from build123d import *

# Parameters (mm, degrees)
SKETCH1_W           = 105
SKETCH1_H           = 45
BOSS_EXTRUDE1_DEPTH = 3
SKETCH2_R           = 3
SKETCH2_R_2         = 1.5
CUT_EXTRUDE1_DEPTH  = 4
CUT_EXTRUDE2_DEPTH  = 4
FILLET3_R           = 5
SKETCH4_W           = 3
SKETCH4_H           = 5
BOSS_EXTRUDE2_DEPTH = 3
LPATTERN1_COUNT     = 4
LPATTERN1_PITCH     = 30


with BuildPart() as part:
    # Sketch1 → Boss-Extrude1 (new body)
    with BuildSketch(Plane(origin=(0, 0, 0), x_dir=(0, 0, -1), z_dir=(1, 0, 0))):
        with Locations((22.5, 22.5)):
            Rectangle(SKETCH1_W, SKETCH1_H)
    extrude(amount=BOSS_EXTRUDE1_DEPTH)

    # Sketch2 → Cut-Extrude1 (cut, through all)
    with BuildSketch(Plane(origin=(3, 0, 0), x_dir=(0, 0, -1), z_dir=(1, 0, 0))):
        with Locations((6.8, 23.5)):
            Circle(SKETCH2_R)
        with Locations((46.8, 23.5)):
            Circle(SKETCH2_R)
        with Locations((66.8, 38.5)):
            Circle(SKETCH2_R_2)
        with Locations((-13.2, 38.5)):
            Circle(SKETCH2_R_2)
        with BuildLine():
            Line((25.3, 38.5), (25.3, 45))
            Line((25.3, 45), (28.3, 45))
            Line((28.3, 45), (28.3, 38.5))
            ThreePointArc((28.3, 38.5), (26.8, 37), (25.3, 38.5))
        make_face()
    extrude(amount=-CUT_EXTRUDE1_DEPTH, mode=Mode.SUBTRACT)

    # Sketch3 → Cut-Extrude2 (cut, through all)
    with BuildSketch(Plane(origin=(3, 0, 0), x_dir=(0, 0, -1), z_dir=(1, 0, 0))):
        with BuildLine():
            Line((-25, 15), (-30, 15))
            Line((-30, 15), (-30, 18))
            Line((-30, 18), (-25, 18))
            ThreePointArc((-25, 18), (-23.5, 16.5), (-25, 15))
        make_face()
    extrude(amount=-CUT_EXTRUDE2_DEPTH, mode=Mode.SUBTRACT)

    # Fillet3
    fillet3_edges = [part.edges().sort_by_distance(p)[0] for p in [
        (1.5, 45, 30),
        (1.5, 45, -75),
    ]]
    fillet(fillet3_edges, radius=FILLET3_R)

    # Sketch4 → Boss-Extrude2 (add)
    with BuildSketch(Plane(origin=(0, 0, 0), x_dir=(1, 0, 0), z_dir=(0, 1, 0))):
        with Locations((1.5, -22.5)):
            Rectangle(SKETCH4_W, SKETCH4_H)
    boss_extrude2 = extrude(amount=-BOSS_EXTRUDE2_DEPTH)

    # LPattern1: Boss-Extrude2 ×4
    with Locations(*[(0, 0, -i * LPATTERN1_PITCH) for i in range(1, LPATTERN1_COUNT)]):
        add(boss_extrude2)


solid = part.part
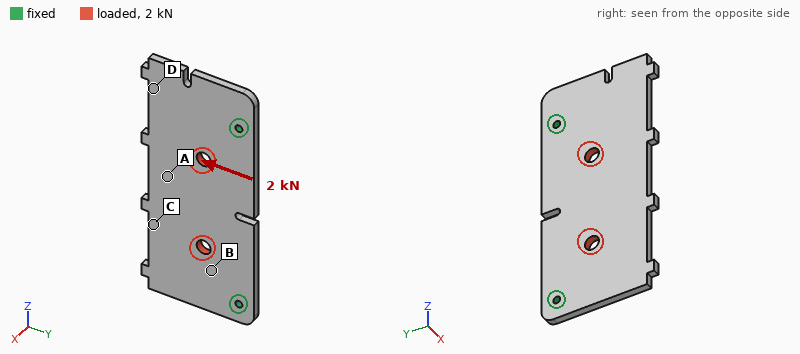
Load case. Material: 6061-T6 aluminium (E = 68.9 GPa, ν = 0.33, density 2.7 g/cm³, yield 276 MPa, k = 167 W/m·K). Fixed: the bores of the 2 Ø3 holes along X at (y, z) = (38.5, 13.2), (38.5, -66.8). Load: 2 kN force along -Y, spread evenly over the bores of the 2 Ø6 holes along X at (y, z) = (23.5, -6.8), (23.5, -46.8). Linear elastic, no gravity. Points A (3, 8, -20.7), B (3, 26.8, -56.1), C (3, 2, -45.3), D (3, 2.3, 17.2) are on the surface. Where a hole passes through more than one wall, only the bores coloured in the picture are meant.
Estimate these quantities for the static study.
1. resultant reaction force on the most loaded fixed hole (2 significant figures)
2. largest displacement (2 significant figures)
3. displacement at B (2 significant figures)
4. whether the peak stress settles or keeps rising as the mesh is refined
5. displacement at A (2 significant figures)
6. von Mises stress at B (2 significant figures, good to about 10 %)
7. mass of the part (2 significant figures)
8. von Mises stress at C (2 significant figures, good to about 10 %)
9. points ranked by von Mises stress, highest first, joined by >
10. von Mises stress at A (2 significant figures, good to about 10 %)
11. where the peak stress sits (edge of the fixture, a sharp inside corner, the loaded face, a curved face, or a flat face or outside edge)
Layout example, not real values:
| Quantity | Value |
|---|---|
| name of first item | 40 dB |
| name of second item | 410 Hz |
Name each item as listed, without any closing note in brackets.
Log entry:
| Quantity | Value |
|---|---|
| resultant reaction force on the most loaded fixed hole | 1.2 kN |
| largest displacement | 18 µm |
| displacement at B | 8.9 µm |
| whether the peak stress settles or keeps rising as the mesh is refined | keeps rising |
| displacement at A | 16 µm |
| von Mises stress at B | 20 MPa |
| mass of the part | 38 g |
| von Mises stress at C | 14 MPa |
| points ranked by von Mises stress, highest first, joined by > | B > C > A > D |
| von Mises stress at A | 11 MPa |
| where the peak stress sits | edge of the fixture |
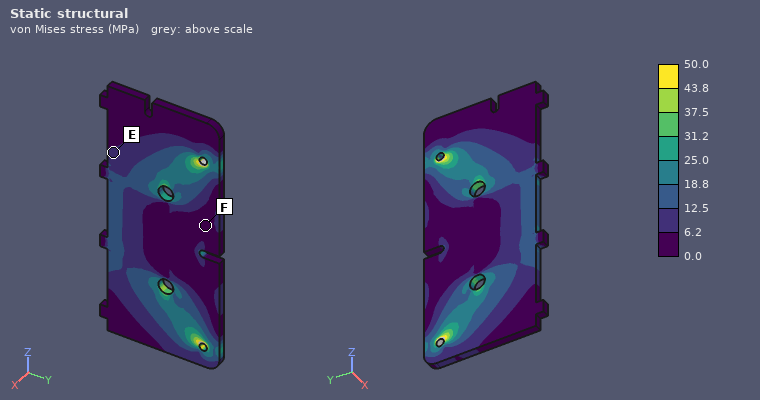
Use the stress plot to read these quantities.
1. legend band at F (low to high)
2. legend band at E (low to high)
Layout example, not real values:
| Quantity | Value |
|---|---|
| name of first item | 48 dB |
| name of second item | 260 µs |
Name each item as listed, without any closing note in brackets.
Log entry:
| Quantity | Value |
|---|---|
| legend band at F | 0.0 to 6.2 MPa |
| legend band at E | 6.2 to 12.5 MPa |
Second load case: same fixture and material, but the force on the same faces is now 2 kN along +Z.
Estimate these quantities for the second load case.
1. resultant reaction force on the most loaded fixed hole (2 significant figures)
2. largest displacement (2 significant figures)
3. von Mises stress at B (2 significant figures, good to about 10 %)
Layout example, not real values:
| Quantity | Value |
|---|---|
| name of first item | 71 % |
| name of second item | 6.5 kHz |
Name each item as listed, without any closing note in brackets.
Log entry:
| Quantity | Value |
|---|---|
| resultant reaction force on the most loaded fixed hole | 1.1 kN |
| largest displacement | 12 µm |
| von Mises stress at B | 16 MPa |
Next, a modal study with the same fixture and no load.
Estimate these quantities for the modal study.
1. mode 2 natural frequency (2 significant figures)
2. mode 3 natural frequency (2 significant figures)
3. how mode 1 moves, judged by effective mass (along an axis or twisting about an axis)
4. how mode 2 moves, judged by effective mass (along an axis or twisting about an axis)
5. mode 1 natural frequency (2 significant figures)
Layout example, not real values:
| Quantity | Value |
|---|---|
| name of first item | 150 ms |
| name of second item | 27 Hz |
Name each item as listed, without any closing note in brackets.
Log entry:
| Quantity | Value |
|---|---|
| mode 2 natural frequency | 1800 Hz |
| mode 3 natural frequency | 2300 Hz |
| how mode 1 moves, judged by effective mass | along X |
| how mode 2 moves, judged by effective mass | twisting about Y |
| mode 1 natural frequency | 1000 Hz |
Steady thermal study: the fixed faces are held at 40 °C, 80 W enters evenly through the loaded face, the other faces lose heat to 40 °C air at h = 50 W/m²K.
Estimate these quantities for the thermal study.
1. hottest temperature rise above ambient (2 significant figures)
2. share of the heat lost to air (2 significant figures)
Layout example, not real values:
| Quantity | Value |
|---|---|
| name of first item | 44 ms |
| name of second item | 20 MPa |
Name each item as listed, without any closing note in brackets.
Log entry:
| Quantity | Value |
|---|---|
| hottest temperature rise above ambient | 71 K |
| share of the heat lost to air | 26 % |
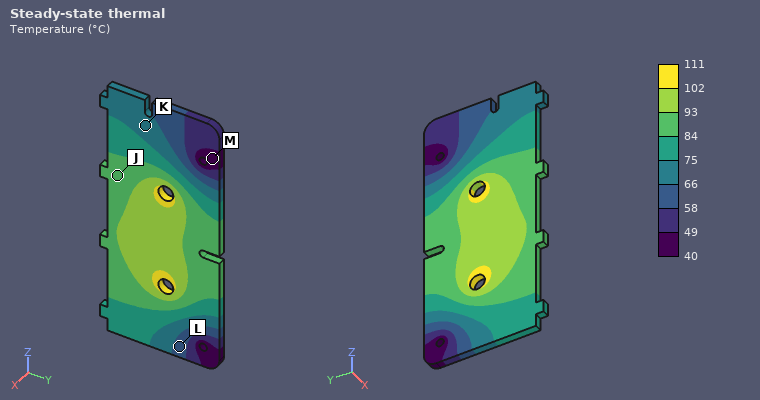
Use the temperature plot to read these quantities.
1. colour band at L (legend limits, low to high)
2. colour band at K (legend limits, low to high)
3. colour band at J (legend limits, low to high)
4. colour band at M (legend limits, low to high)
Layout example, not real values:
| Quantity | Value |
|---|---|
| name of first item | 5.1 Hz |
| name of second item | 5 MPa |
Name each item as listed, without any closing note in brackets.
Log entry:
| Quantity | Value |
|---|---|
| colour band at L | 58 to 66 °C |
| colour band at K | 66 to 75 °C |
| colour band at J | 84 to 93 °C |
| colour band at M | 40 to 49 °C |
